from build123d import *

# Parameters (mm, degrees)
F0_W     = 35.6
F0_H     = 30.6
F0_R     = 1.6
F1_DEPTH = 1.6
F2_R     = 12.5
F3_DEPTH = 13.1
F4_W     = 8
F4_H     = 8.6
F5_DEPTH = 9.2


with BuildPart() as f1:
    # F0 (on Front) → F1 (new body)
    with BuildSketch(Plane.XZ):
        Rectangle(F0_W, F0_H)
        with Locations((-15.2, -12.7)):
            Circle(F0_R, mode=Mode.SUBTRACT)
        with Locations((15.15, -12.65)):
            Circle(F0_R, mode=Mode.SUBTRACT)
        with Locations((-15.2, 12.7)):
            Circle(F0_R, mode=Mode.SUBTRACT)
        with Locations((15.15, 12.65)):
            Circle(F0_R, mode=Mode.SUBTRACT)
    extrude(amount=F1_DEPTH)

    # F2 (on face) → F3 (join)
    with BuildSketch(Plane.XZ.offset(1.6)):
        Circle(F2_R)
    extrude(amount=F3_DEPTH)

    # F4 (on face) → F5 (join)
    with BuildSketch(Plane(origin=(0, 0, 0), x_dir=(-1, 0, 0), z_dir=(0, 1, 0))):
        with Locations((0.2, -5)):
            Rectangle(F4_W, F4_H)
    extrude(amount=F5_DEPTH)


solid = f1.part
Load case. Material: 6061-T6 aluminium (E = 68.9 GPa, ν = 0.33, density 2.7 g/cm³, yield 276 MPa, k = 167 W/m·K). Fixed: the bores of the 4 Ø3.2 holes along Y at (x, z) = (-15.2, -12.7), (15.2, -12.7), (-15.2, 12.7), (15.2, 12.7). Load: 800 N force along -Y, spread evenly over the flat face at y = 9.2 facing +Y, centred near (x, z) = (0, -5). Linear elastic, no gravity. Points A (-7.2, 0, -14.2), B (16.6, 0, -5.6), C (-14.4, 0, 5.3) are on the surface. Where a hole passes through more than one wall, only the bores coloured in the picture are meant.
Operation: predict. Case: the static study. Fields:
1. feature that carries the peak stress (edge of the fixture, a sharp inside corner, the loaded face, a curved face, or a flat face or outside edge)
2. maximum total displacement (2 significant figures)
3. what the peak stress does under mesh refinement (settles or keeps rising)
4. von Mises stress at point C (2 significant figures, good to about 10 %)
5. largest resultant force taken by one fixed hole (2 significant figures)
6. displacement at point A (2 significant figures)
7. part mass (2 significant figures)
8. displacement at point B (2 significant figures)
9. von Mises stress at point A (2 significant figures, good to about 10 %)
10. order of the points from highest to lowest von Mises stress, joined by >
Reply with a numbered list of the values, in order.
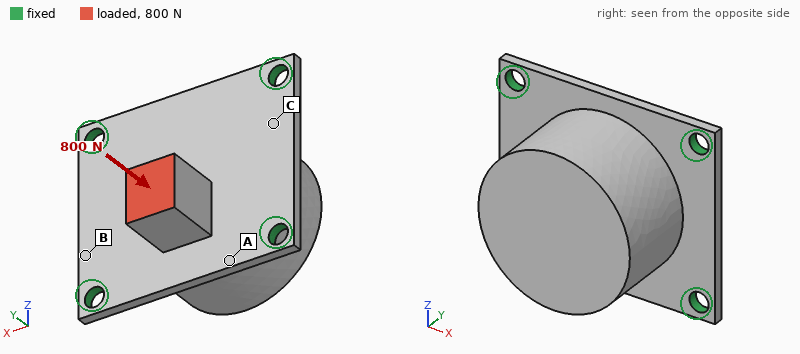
1. edge of the fixture
2. 52 µm
3. keeps rising
4. 18 MPa
5. 310 N
6. 36 µm
7. 24 g
8. 17 µm
9. 67 MPa
10. A > B > C
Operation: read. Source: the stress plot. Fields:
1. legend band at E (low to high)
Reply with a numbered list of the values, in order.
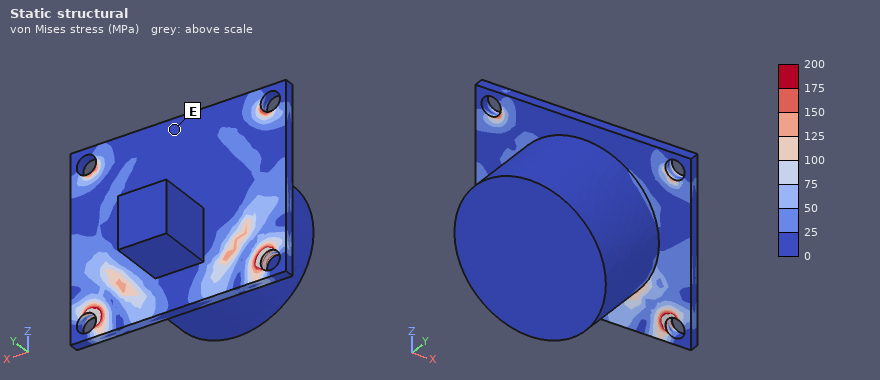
1. 0 to 25 MPa
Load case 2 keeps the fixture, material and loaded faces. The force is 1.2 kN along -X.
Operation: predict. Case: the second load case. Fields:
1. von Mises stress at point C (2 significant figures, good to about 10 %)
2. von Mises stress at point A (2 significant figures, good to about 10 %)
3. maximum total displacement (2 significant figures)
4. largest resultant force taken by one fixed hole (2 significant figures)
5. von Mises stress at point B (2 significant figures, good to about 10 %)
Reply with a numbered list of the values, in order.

1. 64 MPa
2. 78 MPa
3. 70 µm
4. 470 N
5. 32 MPa
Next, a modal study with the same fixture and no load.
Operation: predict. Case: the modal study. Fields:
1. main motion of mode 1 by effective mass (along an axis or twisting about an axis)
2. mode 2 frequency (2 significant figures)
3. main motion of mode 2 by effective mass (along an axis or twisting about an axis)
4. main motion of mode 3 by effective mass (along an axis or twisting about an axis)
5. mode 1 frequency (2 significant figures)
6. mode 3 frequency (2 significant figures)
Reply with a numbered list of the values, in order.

1. along Y
2. 5800 Hz
3. along Z
4. along X
5. 5500 Hz
6. 7000 Hz
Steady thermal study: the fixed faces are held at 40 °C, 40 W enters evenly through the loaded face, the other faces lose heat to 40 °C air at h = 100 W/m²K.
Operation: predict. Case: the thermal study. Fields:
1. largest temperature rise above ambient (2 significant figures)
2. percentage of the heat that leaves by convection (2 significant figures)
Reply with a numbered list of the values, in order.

1. 64 K
2. 19 %
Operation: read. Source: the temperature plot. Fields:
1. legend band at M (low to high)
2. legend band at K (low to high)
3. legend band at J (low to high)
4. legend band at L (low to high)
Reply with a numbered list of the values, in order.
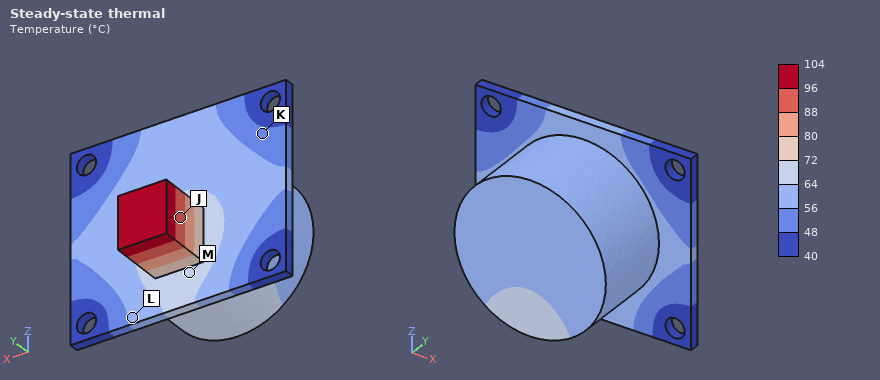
1. 64 to 72 °C
2. 48 to 56 °C
3. 88 to 96 °C
4. 56 to 64 °C
